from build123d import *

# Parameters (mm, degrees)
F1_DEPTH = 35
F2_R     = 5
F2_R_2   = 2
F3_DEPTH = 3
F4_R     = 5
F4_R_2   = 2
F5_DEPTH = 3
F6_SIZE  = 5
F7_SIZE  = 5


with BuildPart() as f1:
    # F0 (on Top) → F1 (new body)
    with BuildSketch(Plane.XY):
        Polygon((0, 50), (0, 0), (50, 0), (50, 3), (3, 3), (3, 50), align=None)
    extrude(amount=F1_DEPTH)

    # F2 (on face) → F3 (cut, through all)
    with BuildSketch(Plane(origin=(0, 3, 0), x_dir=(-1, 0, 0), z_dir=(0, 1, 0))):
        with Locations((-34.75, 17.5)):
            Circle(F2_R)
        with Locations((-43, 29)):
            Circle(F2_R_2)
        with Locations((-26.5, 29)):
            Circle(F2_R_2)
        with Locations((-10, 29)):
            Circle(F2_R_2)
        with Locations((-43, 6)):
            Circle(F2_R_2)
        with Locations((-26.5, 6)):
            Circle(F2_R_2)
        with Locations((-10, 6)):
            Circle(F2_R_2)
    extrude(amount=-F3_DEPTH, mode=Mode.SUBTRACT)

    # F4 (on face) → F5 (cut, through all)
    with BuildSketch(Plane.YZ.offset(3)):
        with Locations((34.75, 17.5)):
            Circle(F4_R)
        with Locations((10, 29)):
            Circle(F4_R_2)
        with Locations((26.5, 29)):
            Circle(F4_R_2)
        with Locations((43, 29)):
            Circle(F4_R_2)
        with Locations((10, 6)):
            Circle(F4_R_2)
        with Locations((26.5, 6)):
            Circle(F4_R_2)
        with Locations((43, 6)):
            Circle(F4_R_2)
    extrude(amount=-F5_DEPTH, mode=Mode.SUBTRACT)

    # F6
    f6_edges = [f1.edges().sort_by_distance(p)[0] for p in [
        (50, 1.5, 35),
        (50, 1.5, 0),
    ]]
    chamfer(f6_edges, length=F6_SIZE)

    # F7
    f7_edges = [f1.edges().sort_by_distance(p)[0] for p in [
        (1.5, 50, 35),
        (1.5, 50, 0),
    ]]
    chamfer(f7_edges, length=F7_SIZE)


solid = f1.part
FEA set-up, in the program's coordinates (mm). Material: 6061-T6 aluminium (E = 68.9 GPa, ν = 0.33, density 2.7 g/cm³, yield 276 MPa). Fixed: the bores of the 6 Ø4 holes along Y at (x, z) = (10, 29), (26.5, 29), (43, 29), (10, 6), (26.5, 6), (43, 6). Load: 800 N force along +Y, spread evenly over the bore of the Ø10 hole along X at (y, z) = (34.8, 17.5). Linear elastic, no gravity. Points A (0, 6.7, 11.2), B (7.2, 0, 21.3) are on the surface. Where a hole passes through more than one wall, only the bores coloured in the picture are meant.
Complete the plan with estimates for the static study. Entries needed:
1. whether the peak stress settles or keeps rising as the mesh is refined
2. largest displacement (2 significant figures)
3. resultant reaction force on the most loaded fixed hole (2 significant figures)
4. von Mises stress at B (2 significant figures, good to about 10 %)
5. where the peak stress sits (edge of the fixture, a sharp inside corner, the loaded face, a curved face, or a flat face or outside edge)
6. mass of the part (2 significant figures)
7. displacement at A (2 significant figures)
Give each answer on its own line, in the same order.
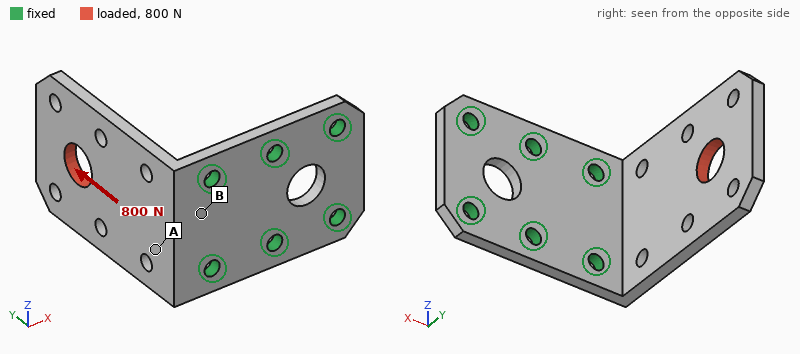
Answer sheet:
keeps rising
0.23 mm
440 N
42 MPa
edge of the fixture
25 g
0.044 mm
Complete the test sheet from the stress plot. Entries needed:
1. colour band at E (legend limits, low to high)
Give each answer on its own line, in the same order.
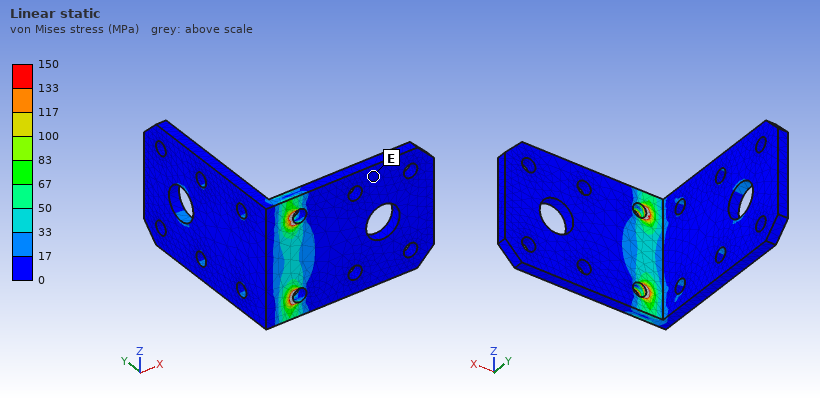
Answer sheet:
0 to 17 MPa
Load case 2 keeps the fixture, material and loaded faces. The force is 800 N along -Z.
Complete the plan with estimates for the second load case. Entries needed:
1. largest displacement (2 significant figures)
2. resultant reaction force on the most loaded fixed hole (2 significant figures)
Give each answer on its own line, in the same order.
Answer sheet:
0.27 mm
1.2 kN
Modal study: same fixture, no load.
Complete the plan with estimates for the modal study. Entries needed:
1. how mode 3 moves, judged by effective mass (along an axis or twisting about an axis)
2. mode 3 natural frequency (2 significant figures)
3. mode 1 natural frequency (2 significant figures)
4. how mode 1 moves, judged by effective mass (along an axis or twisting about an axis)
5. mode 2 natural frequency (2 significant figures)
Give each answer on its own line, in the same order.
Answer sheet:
along Z
3900 Hz
900 Hz
along X
2900 Hz
